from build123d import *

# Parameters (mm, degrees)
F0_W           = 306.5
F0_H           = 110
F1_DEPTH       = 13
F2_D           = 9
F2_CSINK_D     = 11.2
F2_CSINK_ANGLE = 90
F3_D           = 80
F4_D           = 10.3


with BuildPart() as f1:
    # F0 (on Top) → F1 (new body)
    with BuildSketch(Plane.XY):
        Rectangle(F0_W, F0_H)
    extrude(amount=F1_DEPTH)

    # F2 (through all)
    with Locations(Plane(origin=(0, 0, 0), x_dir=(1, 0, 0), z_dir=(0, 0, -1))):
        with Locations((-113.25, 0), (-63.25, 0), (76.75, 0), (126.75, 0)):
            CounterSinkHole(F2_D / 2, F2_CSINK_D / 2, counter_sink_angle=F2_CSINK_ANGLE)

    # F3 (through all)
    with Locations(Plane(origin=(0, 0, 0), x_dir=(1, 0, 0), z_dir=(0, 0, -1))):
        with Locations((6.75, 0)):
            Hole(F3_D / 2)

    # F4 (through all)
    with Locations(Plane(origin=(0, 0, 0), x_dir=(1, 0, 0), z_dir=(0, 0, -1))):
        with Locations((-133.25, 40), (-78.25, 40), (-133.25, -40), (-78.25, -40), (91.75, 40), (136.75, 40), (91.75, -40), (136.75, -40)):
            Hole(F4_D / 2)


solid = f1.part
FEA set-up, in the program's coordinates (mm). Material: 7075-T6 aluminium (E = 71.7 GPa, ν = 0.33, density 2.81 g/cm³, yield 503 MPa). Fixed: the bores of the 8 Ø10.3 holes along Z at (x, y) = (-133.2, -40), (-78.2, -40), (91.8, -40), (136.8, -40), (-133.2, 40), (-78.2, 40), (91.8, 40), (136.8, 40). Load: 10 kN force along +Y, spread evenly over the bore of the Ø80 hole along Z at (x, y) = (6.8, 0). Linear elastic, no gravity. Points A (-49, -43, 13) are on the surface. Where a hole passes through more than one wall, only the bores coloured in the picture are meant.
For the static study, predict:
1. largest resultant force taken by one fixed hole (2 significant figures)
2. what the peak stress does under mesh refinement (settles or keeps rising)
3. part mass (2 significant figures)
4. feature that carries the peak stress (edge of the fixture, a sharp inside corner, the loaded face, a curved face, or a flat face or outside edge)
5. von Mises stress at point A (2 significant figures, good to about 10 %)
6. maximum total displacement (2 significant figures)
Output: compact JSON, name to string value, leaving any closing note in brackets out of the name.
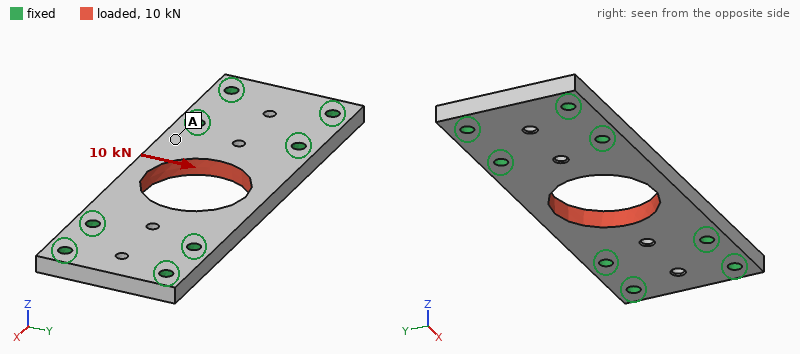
{"largest resultant force taken by one fixed hole": "3.0 kN", "what the peak stress does under mesh refinement": "keeps rising", "part mass": "1.0 kg", "feature that carries the peak stress": "edge of the fixture", "von Mises stress at point A": "2.6 MPa", "maximum total displacement": "21 µm"}
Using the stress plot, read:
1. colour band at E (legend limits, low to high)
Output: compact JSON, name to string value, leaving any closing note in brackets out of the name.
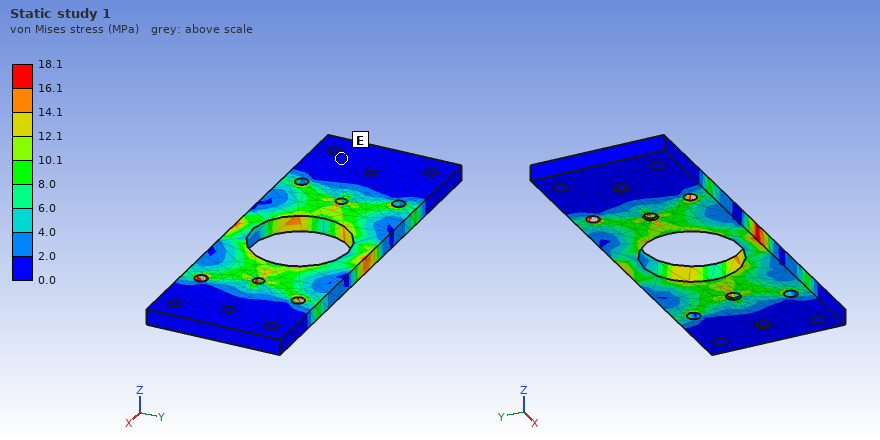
{"colour band at E": "0.0 to 2.0 MPa"}
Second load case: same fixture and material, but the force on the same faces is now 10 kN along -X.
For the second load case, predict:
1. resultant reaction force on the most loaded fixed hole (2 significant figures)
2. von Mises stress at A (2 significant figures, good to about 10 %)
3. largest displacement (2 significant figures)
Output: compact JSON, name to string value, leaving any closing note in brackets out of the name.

{"resultant reaction force on the most loaded fixed hole": "2.1 kN", "von Mises stress at A": "4.2 MPa", "largest displacement": "4.7 µm"}
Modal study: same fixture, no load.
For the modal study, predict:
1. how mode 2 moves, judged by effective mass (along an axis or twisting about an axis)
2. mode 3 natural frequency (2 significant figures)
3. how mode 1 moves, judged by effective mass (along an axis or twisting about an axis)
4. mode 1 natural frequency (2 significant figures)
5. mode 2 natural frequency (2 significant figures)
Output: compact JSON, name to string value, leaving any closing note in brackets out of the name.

{"how mode 2 moves, judged by effective mass": "twisting about X", "mode 3 natural frequency": "5000 Hz", "how mode 1 moves, judged by effective mass": "along Z", "mode 1 natural frequency": "2700 Hz", "mode 2 natural frequency": "3200 Hz"}
